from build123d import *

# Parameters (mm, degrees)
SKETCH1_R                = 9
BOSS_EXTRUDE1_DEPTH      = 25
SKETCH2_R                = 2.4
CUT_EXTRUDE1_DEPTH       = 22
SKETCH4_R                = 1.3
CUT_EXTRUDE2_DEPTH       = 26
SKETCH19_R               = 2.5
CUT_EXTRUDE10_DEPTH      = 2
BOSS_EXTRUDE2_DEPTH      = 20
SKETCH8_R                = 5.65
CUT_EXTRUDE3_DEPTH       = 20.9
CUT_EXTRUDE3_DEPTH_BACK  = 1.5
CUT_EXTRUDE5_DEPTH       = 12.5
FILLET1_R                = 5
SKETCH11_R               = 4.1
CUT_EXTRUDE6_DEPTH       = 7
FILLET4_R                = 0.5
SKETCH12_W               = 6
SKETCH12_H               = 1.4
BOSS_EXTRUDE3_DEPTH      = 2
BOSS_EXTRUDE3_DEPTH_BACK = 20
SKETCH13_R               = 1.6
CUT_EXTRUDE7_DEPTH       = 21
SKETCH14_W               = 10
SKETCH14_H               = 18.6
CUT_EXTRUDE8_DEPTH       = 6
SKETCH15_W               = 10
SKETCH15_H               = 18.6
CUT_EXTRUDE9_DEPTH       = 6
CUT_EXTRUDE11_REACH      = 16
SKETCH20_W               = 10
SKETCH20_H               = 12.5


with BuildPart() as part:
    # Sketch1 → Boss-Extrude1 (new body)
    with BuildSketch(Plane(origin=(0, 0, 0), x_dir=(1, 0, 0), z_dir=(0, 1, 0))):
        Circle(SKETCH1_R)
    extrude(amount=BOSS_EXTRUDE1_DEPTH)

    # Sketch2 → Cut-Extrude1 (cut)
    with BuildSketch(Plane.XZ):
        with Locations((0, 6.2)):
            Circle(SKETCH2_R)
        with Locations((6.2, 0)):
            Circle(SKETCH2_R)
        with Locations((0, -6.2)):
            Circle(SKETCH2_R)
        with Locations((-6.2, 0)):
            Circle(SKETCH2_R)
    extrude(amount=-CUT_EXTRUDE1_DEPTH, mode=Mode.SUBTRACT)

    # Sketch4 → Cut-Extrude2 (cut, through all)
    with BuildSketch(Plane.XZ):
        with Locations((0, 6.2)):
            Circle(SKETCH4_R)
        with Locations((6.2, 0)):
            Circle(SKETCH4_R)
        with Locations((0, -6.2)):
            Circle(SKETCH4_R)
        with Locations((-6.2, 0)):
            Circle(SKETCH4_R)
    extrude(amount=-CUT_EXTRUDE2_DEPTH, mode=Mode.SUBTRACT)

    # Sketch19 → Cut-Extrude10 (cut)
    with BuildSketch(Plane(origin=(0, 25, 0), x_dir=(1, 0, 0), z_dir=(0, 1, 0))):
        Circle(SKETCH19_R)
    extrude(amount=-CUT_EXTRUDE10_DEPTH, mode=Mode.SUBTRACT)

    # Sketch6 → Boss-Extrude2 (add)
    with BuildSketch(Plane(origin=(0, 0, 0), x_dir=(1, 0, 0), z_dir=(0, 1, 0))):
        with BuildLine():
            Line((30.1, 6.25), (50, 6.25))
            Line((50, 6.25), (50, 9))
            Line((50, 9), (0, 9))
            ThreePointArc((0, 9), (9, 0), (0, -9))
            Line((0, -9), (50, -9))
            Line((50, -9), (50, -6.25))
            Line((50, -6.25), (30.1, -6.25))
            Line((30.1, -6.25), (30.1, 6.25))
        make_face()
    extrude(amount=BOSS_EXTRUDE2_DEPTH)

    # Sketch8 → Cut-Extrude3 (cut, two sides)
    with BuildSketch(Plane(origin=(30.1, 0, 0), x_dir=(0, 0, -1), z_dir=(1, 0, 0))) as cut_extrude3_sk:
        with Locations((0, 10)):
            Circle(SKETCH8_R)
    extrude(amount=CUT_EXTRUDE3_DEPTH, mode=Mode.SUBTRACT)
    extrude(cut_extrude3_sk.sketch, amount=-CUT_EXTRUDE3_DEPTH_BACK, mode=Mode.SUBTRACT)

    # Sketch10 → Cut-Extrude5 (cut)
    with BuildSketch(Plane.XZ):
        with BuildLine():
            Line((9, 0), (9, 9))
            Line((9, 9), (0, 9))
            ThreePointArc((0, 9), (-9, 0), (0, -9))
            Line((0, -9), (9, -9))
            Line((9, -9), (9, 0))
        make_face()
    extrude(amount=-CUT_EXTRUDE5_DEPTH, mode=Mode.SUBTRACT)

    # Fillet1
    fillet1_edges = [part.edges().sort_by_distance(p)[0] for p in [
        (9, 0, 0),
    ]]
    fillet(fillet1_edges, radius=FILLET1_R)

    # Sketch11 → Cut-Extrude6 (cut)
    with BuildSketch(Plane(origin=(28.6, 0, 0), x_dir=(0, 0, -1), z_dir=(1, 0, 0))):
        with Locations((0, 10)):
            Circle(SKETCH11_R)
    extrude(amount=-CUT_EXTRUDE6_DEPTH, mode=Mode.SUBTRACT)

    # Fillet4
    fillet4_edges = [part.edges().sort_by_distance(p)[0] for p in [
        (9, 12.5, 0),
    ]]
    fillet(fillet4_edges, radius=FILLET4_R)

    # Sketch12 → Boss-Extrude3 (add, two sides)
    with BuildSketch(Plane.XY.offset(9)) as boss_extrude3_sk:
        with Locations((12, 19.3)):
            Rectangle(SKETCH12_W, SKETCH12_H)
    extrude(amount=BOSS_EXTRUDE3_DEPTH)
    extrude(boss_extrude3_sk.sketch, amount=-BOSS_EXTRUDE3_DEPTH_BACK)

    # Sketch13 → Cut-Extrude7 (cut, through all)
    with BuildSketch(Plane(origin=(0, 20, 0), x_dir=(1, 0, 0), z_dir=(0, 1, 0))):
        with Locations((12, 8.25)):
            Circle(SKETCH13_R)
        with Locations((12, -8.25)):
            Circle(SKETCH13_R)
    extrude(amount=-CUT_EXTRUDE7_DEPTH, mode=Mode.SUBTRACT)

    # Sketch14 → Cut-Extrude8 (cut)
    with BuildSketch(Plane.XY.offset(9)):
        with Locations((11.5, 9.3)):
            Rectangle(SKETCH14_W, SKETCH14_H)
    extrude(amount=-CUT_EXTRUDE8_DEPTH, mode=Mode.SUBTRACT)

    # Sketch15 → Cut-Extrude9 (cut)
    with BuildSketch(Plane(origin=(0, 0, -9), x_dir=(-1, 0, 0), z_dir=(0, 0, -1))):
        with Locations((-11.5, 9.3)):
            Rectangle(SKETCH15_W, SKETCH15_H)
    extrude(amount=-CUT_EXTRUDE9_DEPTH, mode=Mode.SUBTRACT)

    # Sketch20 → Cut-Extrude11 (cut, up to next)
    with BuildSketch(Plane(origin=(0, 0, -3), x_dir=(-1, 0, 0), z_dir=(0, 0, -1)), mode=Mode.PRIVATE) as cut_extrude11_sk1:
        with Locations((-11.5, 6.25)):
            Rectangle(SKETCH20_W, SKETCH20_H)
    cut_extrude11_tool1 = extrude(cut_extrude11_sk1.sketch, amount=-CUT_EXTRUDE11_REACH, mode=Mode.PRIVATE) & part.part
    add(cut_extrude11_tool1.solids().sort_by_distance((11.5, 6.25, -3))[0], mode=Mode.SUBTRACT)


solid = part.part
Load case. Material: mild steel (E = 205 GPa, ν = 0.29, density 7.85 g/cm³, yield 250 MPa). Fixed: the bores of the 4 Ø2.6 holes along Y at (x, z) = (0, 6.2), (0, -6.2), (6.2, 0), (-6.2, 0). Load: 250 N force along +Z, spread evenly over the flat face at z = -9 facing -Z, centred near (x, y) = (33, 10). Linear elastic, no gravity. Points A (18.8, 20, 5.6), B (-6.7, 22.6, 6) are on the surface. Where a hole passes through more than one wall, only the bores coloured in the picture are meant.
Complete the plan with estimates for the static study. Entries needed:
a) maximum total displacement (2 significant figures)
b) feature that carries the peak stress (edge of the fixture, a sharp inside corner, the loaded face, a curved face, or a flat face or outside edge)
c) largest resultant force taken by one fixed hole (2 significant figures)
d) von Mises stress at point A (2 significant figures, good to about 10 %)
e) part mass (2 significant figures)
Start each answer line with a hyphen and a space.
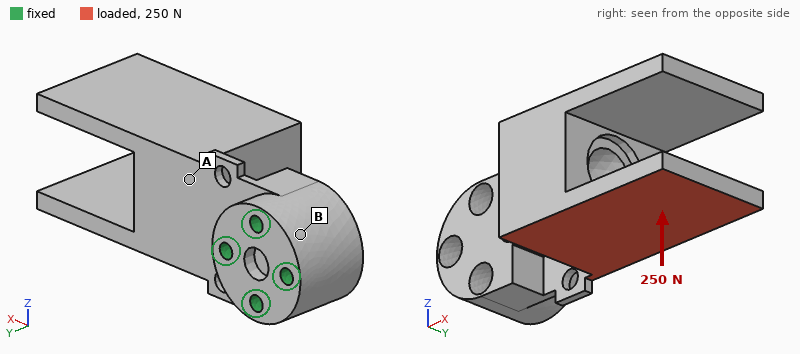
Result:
- 75 µm
- a curved face
- 450 N
- 20 MPa
- 75 g
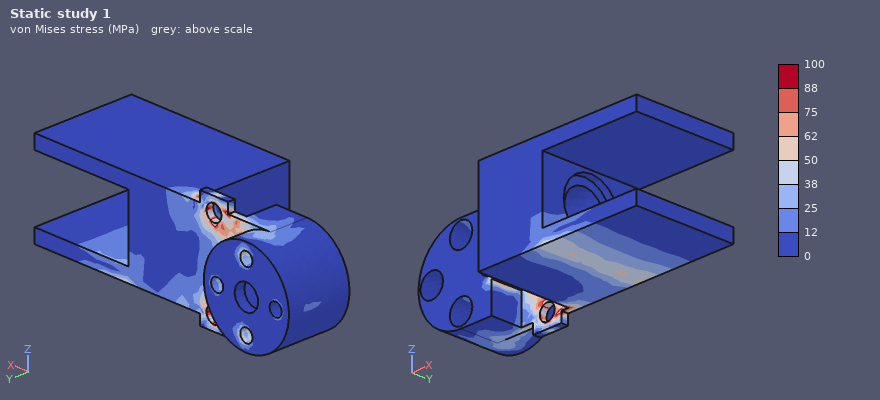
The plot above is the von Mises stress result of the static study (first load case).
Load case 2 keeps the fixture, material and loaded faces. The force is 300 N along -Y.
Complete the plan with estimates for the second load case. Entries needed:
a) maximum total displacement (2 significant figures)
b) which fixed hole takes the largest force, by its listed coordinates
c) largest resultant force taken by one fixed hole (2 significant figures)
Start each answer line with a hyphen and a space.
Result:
- 0.12 mm
- (6.2, 0)
- 820 N
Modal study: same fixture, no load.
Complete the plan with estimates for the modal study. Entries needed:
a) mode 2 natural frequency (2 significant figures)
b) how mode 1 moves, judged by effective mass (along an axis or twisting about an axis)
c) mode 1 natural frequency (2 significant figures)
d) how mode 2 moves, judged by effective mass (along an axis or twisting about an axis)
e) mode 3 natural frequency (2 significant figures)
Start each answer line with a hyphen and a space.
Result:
- 2100 Hz
- along Y
- 1700 Hz
- along Z
- 3700 Hz
